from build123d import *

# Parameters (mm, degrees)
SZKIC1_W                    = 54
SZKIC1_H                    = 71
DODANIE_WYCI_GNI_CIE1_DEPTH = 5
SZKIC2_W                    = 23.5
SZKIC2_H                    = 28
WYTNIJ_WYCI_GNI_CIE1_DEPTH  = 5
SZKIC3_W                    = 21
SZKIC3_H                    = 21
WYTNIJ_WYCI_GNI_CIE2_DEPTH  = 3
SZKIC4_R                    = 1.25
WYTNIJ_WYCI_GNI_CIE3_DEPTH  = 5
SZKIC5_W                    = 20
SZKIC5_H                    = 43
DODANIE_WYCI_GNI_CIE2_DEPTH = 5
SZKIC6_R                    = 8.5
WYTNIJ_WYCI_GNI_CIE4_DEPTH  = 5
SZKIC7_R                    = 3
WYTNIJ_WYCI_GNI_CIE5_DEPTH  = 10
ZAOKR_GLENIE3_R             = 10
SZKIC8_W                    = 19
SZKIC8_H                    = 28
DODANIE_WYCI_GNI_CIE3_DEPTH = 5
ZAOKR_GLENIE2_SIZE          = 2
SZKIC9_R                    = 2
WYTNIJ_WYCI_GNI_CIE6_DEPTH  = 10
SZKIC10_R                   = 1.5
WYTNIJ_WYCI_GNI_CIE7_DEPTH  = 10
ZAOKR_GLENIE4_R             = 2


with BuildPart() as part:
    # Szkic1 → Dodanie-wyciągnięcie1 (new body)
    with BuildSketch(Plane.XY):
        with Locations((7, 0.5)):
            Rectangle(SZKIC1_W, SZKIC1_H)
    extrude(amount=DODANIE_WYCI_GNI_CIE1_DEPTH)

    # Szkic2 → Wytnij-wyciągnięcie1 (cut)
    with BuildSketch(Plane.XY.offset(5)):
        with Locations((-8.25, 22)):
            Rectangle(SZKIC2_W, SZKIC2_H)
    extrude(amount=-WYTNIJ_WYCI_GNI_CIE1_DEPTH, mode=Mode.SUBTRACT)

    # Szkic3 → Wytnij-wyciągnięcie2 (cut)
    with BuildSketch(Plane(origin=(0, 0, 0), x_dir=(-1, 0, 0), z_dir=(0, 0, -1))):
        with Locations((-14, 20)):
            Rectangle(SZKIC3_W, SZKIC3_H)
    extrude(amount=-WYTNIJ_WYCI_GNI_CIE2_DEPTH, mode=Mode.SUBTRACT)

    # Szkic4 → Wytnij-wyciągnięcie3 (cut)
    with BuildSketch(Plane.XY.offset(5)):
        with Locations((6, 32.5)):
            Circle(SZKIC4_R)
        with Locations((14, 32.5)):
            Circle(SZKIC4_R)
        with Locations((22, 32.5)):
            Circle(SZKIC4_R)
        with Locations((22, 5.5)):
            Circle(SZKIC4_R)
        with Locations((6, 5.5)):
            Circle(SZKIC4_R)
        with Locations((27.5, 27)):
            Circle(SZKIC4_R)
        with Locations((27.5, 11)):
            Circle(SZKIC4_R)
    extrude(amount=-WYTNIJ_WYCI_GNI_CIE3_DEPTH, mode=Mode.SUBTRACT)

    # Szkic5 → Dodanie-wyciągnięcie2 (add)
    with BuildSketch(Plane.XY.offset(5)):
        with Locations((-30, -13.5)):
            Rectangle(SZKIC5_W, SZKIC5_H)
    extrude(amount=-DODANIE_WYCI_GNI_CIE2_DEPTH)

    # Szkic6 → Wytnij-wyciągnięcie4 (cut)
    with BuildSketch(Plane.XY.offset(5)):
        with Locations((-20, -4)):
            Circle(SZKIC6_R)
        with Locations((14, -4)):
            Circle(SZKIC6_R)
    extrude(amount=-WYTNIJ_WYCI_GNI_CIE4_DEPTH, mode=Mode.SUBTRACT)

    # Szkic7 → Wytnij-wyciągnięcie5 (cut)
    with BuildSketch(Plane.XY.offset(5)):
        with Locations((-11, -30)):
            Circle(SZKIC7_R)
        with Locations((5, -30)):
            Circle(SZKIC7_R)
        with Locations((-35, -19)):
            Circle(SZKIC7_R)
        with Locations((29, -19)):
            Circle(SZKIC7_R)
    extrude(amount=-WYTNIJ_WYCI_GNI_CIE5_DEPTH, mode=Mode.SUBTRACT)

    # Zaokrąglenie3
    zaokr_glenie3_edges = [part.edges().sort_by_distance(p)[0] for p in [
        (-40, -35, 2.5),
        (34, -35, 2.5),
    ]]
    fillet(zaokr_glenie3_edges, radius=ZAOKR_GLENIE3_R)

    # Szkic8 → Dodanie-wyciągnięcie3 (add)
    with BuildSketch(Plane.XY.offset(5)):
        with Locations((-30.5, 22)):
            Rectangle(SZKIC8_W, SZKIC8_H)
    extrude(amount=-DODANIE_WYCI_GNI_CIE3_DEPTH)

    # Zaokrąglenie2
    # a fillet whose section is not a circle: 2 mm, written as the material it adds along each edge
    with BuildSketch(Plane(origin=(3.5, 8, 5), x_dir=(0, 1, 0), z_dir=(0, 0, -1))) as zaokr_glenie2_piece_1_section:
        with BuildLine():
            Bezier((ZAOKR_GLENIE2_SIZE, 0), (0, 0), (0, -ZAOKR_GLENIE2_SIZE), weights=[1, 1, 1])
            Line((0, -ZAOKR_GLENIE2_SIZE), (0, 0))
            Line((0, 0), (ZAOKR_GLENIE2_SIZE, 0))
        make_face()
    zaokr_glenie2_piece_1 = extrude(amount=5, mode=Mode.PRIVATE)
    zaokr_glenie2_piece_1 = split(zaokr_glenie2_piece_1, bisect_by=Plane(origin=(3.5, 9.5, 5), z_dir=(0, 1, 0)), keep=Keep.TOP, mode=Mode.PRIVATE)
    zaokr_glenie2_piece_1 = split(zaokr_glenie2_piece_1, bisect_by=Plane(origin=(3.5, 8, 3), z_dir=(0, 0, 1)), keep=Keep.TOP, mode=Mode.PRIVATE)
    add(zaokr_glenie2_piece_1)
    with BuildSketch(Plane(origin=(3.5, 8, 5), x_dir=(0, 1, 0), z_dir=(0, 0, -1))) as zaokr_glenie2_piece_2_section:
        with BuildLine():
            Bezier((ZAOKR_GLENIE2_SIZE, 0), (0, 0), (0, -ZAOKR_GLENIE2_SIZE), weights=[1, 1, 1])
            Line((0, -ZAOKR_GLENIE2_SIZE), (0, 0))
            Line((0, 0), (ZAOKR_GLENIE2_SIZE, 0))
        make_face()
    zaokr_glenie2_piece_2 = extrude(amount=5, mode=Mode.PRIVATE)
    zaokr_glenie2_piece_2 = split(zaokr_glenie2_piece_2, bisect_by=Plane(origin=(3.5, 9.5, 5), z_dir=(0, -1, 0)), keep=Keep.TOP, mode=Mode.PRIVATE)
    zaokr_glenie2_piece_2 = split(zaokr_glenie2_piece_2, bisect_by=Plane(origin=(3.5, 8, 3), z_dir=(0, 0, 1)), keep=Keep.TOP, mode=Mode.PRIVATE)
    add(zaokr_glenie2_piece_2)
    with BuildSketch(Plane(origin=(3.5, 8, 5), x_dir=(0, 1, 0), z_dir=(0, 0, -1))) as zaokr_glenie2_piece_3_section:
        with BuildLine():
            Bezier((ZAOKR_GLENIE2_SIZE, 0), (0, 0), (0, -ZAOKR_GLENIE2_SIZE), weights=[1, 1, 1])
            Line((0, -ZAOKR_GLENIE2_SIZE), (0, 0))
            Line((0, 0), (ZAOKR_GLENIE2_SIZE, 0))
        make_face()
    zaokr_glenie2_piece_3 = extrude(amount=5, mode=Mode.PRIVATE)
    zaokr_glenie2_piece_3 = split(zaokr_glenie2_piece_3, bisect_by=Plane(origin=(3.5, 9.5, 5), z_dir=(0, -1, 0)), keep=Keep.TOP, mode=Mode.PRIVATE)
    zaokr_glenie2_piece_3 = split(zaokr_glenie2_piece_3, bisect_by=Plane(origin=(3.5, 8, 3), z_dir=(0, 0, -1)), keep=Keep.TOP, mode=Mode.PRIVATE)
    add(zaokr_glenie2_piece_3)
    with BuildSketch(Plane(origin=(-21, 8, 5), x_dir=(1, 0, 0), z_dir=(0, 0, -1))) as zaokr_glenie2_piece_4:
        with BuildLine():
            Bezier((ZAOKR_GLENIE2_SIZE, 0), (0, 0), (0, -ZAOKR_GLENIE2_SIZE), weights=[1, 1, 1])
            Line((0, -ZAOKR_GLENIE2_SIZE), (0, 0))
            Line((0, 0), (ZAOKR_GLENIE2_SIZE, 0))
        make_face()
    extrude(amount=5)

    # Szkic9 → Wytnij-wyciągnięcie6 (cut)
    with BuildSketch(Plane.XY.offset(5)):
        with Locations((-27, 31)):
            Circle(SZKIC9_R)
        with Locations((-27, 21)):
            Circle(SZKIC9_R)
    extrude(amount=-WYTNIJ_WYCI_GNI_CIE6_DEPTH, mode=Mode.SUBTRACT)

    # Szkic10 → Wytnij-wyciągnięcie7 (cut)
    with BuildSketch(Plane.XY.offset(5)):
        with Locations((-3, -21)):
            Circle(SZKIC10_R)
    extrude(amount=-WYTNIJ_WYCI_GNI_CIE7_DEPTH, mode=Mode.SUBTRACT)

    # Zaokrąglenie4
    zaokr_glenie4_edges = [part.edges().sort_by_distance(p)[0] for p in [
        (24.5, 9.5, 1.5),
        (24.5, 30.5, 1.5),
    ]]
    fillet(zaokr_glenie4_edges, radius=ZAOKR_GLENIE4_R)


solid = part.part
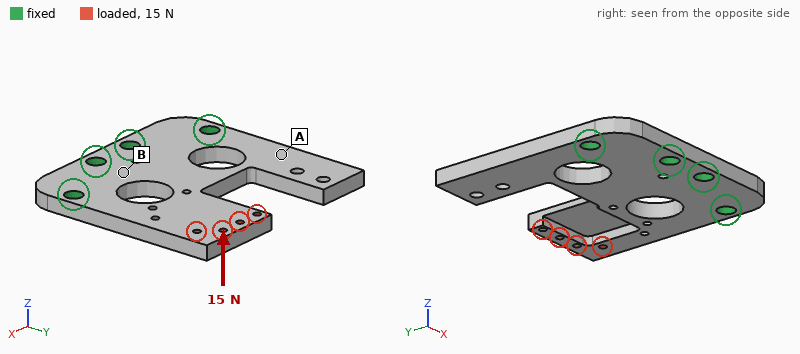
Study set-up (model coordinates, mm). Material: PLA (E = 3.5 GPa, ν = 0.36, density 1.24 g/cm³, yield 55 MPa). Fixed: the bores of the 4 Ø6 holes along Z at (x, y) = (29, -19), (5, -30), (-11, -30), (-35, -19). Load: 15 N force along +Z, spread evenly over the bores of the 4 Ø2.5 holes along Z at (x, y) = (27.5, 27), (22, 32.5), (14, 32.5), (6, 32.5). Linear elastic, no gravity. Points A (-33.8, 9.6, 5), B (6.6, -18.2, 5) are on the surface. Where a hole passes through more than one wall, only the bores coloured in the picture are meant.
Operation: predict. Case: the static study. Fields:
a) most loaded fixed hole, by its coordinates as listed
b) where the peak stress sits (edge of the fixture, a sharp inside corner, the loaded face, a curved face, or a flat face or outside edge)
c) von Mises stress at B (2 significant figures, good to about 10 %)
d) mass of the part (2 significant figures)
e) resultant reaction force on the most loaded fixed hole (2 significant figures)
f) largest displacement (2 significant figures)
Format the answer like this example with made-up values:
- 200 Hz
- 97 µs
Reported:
- (29, -19)
- a curved face
- 1.9 MPa
- 23 g
- 15 N
- 1.0 mm
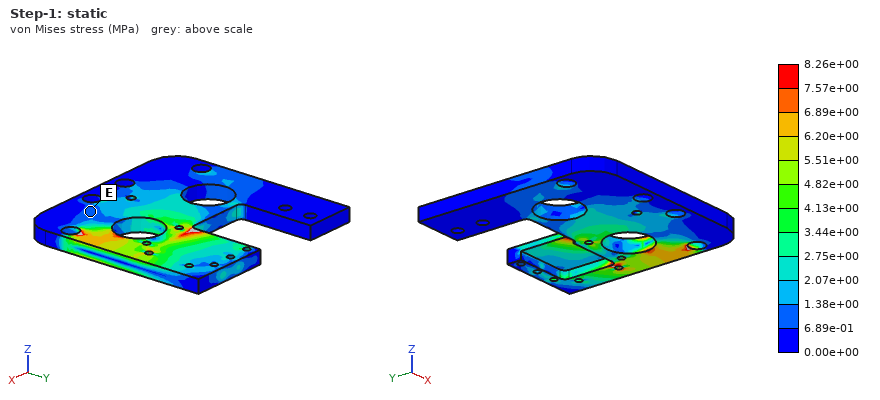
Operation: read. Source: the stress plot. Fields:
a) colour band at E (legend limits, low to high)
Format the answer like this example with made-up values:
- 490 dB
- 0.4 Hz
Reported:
- 6.89e-01 to 1.38e+00 MPa
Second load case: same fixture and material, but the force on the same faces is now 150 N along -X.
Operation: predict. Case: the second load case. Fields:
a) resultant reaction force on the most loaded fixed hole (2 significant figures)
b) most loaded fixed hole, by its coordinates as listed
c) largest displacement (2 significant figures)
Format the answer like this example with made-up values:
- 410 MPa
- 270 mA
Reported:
- 180 N
- (29, -19)
- 0.43 mm
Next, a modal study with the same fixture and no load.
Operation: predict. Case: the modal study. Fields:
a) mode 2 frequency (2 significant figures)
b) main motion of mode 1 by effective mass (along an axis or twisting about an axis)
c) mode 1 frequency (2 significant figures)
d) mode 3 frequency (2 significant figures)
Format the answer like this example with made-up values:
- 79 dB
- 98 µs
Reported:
- 530 Hz
- along Z
- 450 Hz
- 1400 Hz
